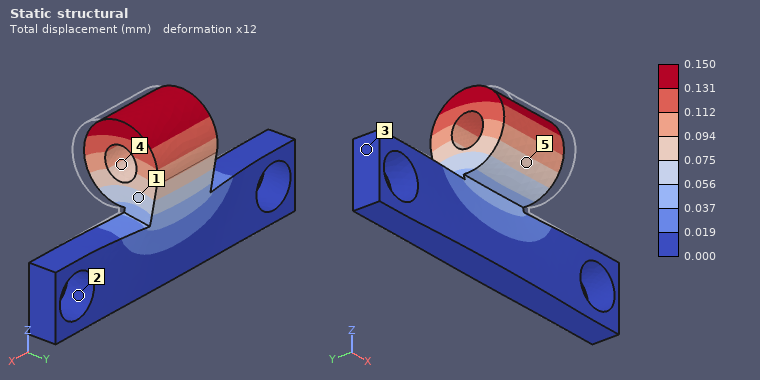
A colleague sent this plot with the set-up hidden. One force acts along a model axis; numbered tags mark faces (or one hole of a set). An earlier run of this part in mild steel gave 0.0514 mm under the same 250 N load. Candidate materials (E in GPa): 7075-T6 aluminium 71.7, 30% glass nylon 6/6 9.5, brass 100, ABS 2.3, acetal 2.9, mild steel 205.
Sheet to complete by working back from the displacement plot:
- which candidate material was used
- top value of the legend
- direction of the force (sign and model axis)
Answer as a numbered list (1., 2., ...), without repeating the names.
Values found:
1. 7075-T6 aluminium
2. 0.150 mm
3. +Y
